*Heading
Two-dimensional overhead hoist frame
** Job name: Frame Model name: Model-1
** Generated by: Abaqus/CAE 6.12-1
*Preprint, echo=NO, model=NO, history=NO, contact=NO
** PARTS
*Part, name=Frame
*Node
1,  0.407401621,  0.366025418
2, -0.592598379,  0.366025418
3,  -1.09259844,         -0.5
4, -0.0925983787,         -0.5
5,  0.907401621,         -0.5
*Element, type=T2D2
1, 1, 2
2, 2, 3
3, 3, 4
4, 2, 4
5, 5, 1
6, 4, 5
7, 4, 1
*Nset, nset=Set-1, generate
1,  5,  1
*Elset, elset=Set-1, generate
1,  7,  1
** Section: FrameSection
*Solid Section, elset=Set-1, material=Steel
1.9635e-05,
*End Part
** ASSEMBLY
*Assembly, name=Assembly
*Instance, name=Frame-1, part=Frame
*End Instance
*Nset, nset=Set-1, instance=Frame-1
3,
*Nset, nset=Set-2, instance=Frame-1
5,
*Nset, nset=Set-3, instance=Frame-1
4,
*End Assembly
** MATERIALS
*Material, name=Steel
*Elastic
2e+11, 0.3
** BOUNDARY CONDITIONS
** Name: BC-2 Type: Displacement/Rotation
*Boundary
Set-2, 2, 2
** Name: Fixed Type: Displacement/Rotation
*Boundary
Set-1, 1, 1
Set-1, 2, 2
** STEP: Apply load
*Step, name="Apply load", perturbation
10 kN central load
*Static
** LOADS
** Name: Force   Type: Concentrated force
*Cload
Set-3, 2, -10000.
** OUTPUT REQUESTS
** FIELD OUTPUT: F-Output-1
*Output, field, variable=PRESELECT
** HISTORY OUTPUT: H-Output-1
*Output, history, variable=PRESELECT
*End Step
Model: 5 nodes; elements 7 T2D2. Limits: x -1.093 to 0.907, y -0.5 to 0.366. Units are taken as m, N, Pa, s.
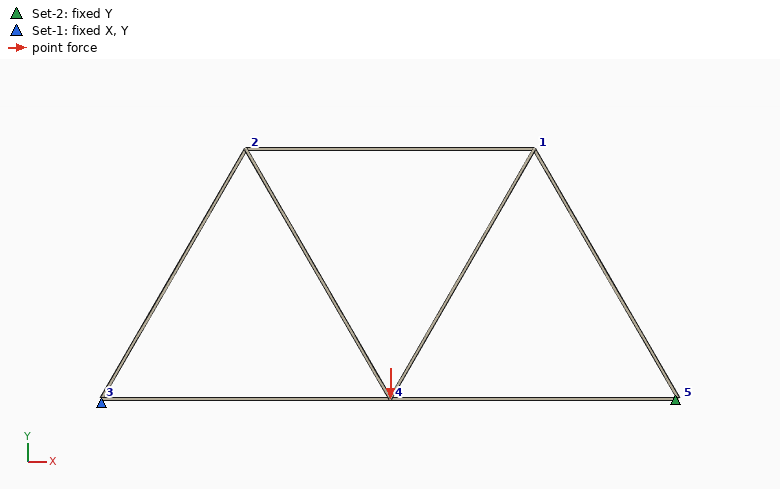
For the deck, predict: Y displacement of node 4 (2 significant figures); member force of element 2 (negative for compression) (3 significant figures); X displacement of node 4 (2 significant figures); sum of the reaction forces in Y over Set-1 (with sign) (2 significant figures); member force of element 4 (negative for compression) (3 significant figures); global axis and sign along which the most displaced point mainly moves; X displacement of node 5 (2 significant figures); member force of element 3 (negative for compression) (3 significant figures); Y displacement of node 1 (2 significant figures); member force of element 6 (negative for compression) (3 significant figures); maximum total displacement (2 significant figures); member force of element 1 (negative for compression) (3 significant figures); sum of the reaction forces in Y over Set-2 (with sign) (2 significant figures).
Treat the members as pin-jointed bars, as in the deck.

-0.0047 m
-5770 N
7.4e-04 m
5000 N
5770 N
-Y
0.0015 m
2890 N
-0.0025 m
2890 N
0.0047 m
-5770 N
5000 N
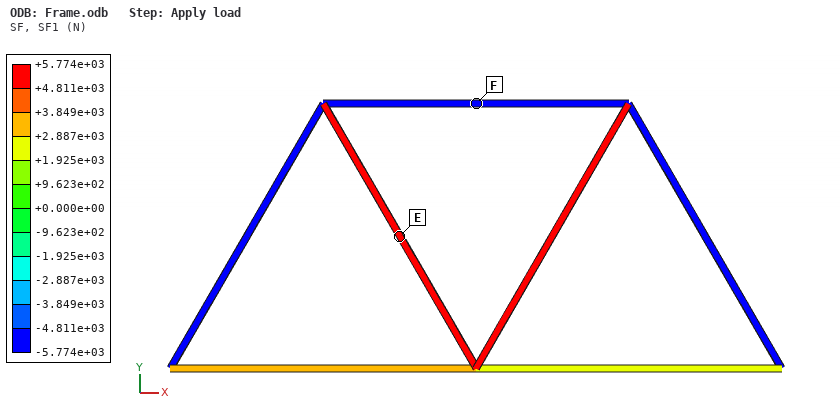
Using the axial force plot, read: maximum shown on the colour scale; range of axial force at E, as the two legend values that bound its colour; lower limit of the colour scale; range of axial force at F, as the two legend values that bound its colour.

+5.774e+03 N
+4.811e+03 to +5.774e+03 N
-5.774e+03 N
-5.774e+03 to -4.811e+03 N
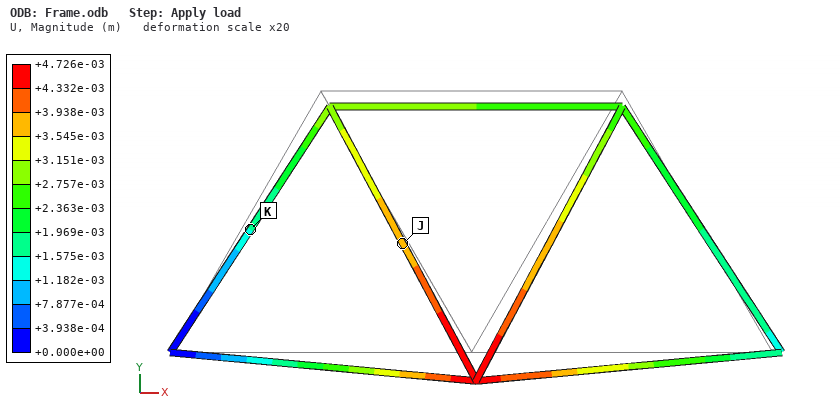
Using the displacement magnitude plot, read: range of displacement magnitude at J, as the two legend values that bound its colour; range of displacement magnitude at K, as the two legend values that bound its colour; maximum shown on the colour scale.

+3.545e-03 to +3.938e-03 m
+1.182e-03 to +1.575e-03 m
+4.726e-03 m
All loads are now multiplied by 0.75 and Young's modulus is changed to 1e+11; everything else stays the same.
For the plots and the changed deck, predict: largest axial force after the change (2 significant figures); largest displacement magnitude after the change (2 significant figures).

4300 N
0.0071 m
